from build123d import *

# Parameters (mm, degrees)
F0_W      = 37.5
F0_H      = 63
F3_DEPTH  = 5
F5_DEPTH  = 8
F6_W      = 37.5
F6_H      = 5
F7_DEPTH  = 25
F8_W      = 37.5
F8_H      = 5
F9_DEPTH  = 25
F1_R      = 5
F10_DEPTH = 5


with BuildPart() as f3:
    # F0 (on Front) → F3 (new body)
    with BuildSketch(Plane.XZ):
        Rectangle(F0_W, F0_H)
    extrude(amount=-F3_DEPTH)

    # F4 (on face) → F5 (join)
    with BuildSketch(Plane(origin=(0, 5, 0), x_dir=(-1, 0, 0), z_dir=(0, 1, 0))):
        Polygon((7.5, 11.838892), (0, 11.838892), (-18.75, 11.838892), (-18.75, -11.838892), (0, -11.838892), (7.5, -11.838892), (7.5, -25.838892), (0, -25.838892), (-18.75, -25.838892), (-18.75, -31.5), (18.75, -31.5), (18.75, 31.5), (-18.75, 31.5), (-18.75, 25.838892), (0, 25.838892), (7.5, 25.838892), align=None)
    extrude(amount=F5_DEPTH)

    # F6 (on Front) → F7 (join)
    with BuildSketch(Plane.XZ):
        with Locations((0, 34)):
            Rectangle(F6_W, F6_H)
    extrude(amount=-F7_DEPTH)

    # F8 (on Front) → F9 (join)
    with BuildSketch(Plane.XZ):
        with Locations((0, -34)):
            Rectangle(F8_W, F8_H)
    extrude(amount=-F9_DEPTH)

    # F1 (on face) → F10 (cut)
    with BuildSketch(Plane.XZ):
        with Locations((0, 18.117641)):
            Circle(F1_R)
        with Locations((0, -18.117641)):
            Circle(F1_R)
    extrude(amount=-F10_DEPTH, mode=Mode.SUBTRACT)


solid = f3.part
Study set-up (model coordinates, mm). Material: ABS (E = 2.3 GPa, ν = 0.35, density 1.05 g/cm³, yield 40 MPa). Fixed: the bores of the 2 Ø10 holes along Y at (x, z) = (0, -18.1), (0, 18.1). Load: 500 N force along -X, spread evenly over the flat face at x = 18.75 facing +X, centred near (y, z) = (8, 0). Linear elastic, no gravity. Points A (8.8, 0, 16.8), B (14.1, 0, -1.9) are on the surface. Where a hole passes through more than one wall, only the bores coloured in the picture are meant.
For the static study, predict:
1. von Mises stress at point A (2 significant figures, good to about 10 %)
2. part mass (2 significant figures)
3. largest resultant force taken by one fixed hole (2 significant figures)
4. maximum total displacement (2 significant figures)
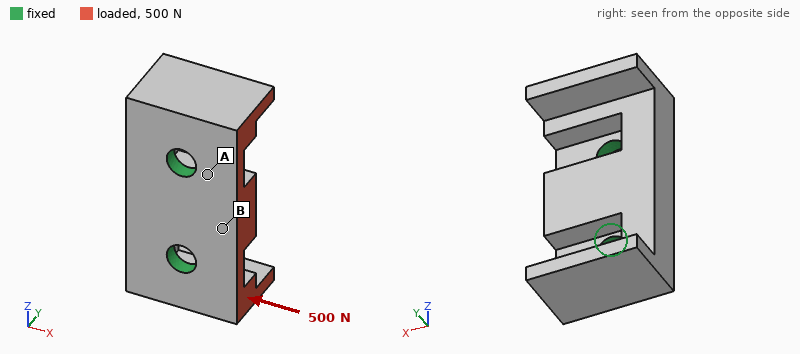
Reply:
1.9 MPa
35 g
250 N
97 µm
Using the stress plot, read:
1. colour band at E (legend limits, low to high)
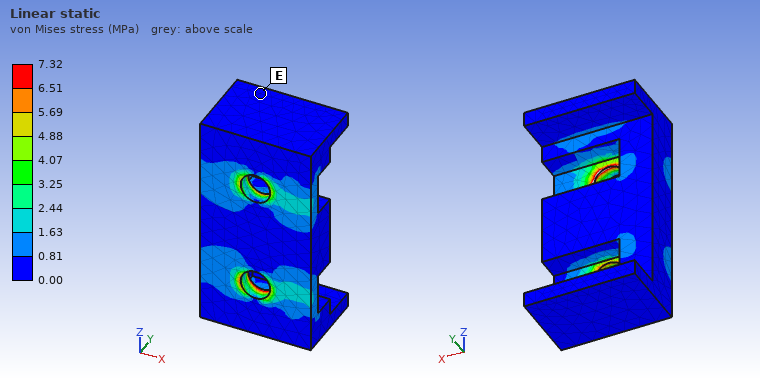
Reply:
0.00 to 0.81 MPa
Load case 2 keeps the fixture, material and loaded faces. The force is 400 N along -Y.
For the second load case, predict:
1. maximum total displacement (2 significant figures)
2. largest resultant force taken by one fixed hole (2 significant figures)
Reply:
0.30 mm
200 N
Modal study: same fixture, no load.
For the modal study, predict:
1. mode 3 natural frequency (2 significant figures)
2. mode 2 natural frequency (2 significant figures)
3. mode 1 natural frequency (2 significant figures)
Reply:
2200 Hz
2100 Hz
2000 Hz
